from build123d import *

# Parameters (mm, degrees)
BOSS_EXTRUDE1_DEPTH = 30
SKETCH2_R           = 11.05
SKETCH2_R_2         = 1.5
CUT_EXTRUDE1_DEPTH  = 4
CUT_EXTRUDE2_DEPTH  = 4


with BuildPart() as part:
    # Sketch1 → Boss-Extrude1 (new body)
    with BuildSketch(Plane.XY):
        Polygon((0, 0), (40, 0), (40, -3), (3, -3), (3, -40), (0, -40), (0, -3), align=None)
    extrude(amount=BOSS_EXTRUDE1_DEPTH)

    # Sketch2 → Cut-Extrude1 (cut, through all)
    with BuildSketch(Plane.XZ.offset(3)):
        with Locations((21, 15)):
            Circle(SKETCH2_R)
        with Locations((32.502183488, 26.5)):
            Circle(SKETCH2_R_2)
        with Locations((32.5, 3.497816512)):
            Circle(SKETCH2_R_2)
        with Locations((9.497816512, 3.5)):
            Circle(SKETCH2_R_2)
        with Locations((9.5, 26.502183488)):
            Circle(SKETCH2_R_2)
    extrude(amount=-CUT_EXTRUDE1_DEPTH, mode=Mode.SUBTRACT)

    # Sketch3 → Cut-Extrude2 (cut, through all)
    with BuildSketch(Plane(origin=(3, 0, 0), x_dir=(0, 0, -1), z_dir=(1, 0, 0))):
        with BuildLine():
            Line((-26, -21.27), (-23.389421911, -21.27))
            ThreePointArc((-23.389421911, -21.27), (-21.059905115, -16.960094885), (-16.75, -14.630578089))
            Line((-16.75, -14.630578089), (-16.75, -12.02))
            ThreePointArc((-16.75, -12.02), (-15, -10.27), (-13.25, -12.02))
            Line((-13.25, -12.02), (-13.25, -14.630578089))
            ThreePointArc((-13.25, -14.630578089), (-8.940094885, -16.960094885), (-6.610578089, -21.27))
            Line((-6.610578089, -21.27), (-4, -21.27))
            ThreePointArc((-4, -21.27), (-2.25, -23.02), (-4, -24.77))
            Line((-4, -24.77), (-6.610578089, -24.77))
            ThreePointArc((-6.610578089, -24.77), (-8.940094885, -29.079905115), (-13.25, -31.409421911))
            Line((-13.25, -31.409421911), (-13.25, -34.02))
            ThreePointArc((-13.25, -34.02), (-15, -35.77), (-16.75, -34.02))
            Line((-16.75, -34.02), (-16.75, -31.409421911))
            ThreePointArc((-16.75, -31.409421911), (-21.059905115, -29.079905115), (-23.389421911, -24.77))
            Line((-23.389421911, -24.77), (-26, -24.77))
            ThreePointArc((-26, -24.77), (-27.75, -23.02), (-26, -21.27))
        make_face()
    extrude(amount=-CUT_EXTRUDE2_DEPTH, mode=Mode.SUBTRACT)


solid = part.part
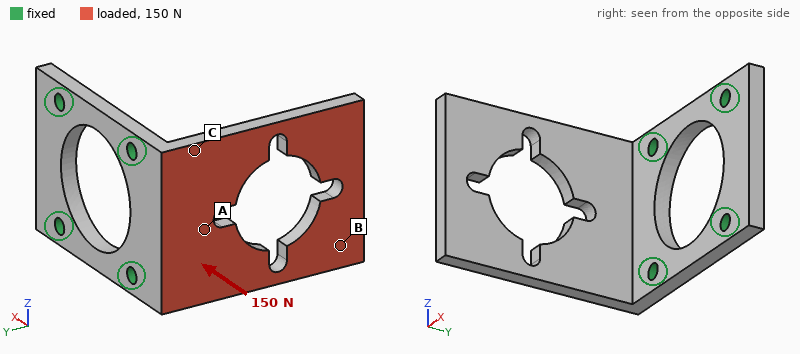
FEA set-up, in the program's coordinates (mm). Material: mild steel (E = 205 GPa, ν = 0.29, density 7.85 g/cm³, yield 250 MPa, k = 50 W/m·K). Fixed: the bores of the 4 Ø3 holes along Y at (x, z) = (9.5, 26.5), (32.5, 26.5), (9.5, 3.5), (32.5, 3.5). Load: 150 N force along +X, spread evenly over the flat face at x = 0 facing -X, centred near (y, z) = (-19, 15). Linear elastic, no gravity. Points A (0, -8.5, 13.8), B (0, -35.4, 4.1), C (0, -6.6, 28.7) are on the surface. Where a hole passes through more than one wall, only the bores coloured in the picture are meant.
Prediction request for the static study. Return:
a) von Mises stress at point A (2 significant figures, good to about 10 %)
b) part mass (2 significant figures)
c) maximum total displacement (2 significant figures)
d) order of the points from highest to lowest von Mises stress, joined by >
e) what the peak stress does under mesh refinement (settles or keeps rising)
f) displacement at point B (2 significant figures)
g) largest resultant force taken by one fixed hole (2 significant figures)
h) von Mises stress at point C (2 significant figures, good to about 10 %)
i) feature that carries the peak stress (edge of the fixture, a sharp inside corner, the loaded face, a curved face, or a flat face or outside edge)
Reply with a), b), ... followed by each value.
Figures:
a) 28 MPa
b) 38 g
c) 0.17 mm
d) C > A > B
e) keeps rising
f) 0.14 mm
g) 83 N
h) 50 MPa
i) edge of the fixture
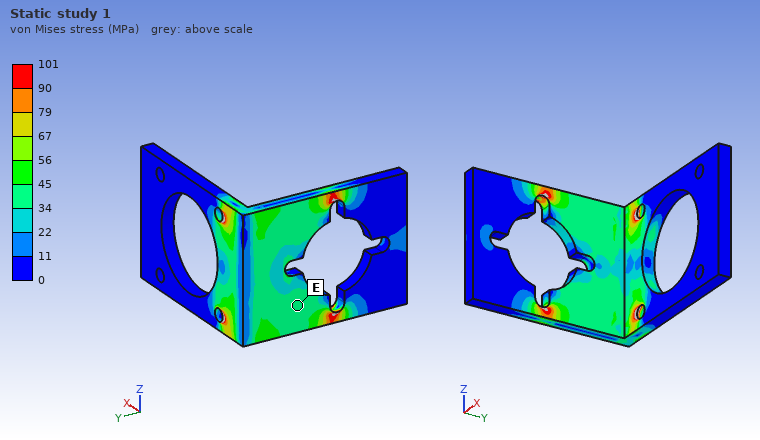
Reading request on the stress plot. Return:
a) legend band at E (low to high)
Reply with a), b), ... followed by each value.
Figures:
a) 34 to 45 MPa
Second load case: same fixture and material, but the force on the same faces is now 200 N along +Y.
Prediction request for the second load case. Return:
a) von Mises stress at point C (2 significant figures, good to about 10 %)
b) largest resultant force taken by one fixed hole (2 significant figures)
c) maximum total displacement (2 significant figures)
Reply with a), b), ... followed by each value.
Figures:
a) 9.0 MPa
b) 100 N
c) 45 µm
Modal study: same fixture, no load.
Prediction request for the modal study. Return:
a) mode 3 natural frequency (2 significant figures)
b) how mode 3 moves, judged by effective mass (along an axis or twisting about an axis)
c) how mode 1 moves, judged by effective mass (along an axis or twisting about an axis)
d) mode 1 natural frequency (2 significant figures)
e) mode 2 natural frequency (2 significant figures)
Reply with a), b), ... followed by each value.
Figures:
a) 4900 Hz
b) along Z
c) along X
d) 1200 Hz
e) 3400 Hz
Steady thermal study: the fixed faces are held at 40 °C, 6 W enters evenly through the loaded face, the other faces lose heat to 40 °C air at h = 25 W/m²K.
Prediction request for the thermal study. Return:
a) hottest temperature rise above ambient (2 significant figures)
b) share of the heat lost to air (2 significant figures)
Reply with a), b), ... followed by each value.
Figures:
a) 45 K
b) 20 %
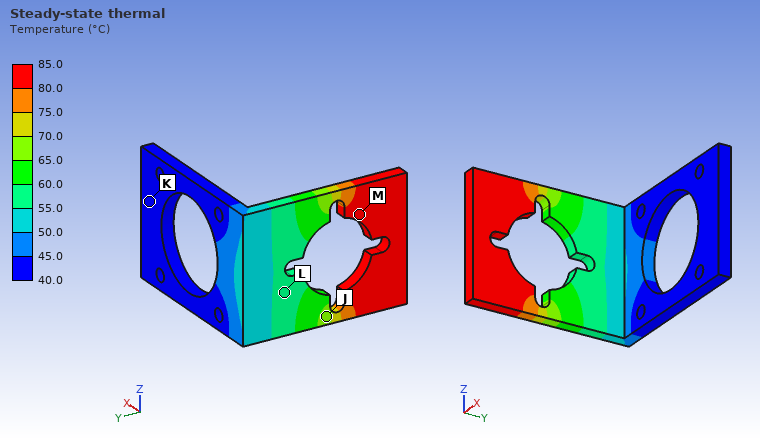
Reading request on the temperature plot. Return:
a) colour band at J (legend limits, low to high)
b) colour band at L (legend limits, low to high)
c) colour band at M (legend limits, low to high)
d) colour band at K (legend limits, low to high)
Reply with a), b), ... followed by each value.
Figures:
a) 65.0 to 70.0 °C
b) 55.0 to 60.0 °C
c) 80.0 to 85.0 °C
d) 40.0 to 45.0 °C
